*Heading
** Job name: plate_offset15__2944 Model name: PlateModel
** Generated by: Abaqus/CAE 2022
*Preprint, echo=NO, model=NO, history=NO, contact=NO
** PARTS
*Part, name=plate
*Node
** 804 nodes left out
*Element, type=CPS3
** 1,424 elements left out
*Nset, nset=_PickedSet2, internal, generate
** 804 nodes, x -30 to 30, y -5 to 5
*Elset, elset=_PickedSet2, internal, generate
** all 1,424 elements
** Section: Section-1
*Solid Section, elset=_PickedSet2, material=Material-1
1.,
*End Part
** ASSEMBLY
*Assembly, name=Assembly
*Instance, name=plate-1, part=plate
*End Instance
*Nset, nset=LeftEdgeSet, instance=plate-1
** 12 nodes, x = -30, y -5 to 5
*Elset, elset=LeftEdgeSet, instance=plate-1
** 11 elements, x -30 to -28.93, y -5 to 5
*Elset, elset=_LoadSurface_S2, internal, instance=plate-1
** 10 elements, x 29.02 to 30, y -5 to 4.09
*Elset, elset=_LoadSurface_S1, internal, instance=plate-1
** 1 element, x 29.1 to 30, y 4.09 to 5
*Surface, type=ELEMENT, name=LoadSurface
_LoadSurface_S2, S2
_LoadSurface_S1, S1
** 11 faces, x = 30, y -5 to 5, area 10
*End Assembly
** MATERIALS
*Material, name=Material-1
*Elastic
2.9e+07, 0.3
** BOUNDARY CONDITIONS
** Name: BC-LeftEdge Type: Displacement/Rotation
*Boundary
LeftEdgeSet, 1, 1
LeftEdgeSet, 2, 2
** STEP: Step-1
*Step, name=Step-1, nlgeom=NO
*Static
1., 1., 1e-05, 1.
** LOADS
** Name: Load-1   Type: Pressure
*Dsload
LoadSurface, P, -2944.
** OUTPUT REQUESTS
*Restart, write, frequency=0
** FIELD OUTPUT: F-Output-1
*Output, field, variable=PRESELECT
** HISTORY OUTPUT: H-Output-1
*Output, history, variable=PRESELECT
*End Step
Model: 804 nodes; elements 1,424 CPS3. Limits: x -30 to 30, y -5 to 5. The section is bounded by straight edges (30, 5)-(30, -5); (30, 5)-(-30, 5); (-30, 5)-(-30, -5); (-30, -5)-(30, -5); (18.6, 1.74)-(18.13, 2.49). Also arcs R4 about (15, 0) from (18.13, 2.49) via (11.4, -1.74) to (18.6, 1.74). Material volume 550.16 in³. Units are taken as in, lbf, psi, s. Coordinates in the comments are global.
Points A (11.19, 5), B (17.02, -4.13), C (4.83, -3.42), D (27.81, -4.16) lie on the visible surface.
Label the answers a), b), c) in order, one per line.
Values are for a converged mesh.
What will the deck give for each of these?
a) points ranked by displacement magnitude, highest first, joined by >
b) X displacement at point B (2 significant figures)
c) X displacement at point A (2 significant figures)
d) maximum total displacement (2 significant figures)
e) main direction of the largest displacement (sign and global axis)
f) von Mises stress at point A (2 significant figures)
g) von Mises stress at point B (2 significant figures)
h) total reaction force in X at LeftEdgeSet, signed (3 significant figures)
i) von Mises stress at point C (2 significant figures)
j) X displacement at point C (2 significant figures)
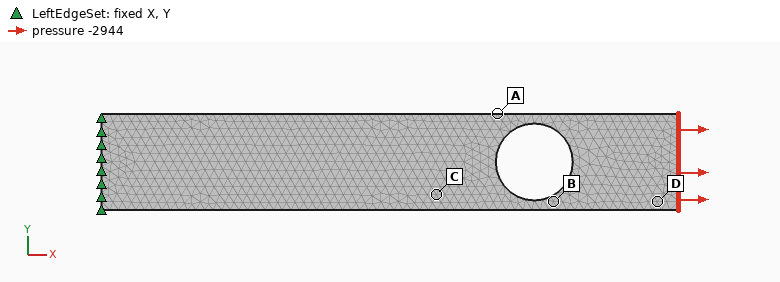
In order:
a) D > B > A > C
b) 0.0076 in
c) 0.0052 in
d) 0.010 in
e) +X
f) 13000 psi
g) 10000 psi
h) -29400 lbf
i) 3400 psi
j) 0.0035 in
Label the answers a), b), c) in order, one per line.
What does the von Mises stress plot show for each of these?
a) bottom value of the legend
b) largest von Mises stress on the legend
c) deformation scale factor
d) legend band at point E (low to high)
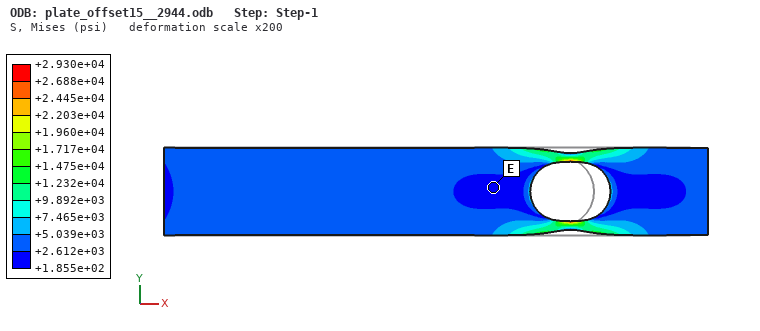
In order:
a) +1.855e+02 psi
b) +2.930e+04 psi
c) 200
d) +1.855e+02 to +2.612e+03 psi
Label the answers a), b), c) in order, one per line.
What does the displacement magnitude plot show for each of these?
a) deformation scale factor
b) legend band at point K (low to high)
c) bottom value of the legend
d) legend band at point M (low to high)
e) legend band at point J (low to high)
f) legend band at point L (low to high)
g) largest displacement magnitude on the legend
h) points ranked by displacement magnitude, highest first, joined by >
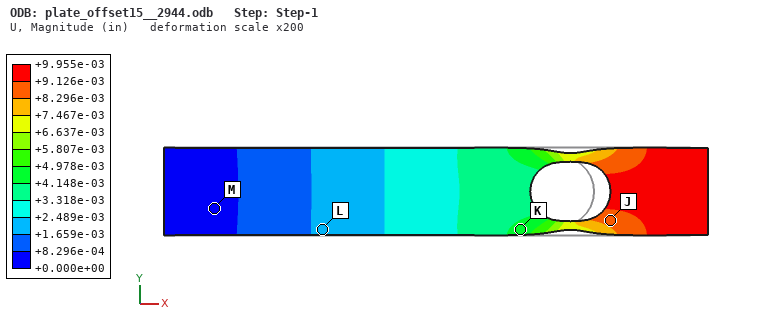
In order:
a) 200
b) +4.148e-03 to +4.978e-03 in
c) +0.000e+00 in
d) +0.000e+00 to +8.296e-04 in
e) +8.296e-03 to +9.126e-03 in
f) +1.659e-03 to +2.489e-03 in
g) +9.955e-03 in
h) J > K > L > M
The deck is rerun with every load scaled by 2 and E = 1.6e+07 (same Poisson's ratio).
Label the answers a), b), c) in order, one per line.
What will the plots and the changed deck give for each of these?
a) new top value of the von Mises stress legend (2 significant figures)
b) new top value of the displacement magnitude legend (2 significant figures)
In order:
a) 59000 psi
b) 0.036 in
